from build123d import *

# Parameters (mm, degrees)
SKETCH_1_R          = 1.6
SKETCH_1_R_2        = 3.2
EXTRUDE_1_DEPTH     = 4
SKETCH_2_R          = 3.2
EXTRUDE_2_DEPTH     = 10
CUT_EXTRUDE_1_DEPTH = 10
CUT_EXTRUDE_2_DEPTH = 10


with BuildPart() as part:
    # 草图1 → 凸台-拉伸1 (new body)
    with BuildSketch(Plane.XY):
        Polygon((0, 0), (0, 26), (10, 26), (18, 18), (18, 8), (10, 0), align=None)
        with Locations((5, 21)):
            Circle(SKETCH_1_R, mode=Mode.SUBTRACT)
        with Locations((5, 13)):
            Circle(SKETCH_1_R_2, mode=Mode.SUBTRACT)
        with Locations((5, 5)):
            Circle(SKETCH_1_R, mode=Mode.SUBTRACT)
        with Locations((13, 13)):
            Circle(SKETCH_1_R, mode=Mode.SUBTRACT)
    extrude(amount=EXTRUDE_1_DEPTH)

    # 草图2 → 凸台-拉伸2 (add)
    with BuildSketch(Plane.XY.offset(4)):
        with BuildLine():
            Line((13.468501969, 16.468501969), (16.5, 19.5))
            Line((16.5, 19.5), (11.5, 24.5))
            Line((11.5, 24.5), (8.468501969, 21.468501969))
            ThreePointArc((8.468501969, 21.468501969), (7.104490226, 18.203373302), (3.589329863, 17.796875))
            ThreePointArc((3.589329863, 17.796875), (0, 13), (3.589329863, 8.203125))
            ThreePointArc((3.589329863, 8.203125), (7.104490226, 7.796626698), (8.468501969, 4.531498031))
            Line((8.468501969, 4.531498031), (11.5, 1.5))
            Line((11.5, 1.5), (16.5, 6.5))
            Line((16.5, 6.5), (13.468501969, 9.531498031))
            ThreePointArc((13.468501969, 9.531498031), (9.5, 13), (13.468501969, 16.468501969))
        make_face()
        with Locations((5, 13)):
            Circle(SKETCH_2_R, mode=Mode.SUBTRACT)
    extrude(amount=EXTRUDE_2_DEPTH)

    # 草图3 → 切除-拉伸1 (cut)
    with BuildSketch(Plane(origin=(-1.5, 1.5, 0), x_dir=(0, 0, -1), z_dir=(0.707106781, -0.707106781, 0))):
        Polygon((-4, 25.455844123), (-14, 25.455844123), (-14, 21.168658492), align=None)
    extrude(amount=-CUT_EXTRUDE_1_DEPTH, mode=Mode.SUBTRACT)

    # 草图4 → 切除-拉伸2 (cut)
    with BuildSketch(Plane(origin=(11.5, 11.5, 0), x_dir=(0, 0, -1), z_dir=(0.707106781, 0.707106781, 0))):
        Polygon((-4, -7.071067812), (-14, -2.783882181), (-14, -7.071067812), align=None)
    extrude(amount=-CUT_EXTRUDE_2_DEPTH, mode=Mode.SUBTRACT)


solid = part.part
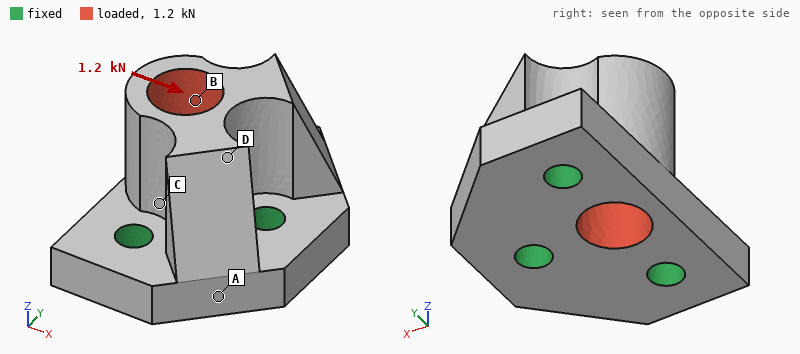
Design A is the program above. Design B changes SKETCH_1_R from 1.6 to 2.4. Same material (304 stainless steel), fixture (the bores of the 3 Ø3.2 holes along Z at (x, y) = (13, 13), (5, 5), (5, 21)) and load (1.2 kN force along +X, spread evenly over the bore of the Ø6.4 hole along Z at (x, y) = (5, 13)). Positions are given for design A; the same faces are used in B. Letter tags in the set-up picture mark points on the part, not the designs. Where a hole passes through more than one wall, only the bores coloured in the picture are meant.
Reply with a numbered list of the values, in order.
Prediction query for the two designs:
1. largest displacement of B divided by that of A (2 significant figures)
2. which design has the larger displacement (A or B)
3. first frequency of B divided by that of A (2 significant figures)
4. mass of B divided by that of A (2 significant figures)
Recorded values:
1. 0.80
2. A
3. 1.2
4. 0.95
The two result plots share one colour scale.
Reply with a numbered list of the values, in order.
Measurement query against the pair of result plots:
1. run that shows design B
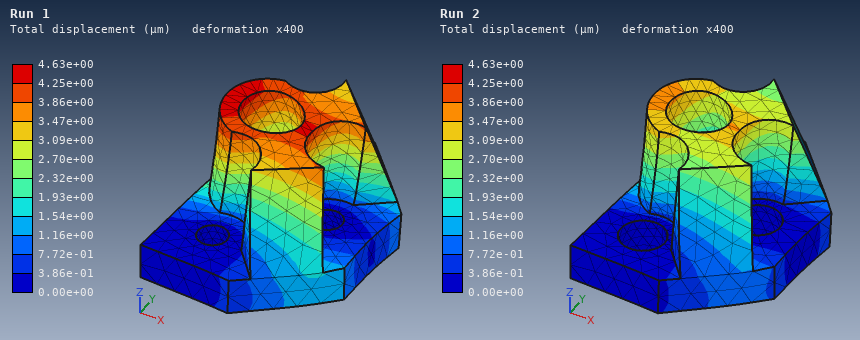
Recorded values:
1. Run 2
